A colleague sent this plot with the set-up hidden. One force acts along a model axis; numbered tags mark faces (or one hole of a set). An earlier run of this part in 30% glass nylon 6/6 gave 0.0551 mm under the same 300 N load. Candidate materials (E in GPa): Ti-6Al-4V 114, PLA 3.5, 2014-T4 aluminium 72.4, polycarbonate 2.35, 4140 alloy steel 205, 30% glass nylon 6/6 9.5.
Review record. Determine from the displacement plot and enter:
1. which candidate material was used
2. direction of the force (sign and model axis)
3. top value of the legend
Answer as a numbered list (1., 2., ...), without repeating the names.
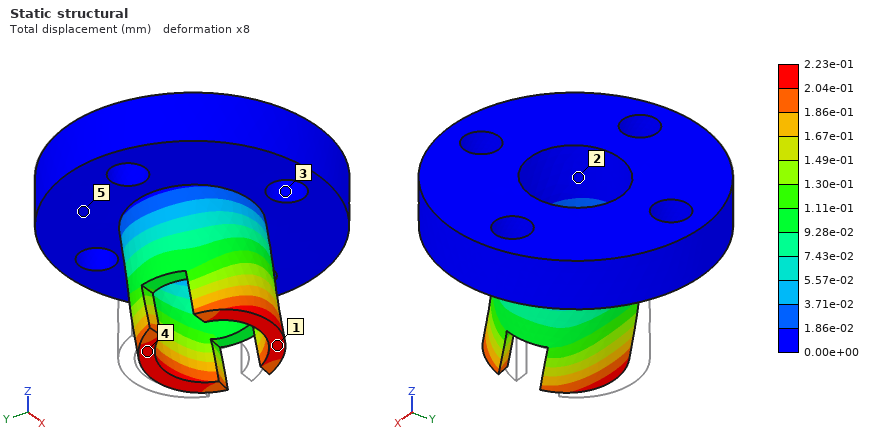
1. polycarbonate
2. -Y
3. 2.23e-01 mm
